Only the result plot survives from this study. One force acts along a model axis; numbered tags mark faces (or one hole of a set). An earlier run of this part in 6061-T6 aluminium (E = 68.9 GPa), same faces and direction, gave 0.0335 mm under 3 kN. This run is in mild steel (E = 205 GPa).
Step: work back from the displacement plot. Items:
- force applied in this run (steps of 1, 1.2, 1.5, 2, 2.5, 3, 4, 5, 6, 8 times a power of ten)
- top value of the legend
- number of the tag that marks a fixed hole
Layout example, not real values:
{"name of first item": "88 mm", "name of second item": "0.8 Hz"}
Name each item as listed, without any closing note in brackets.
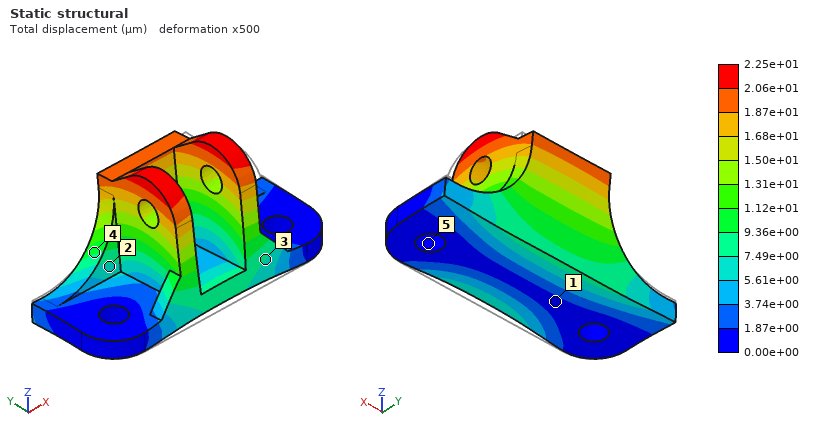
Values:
{"force applied in this run": "6 kN", "top value of the legend": "2.25e+01 µm", "number of the tag that marks a fixed hole": "5"}
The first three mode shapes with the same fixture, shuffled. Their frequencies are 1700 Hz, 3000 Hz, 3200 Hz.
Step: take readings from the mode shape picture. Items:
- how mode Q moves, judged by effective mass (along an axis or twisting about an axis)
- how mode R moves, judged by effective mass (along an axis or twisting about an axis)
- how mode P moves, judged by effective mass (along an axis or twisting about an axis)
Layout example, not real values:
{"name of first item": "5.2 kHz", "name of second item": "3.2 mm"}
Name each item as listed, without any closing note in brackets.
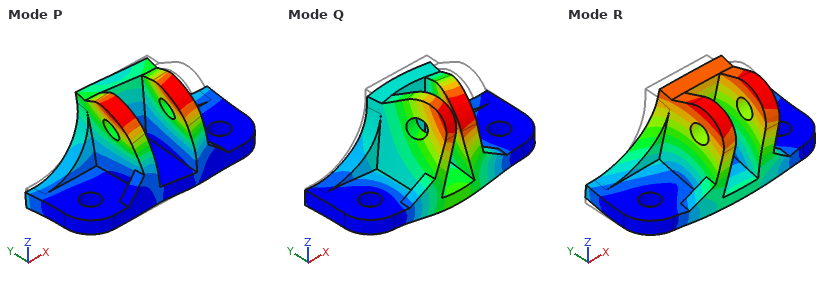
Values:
{"how mode Q moves, judged by effective mass": "along Z", "how mode R moves, judged by effective mass": "along Y", "how mode P moves, judged by effective mass": "along X"}
